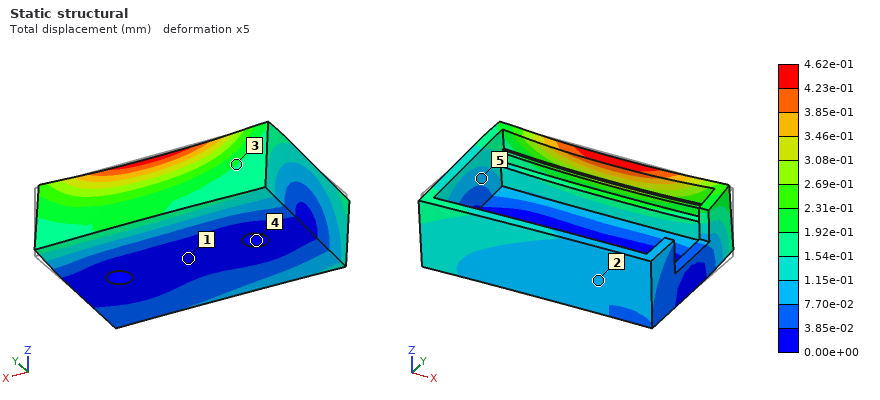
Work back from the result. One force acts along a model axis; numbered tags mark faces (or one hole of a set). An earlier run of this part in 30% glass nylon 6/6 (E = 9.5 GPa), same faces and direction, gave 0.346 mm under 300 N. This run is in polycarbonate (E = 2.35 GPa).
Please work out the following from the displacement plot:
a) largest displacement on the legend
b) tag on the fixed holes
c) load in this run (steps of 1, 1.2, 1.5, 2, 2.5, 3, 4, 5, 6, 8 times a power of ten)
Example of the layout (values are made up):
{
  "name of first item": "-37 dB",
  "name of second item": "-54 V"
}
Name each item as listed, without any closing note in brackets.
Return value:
{
  "largest displacement on the legend": "4.62e-01 mm",
  "tag on the fixed holes": "4",
  "load in this run": "100 N"
}
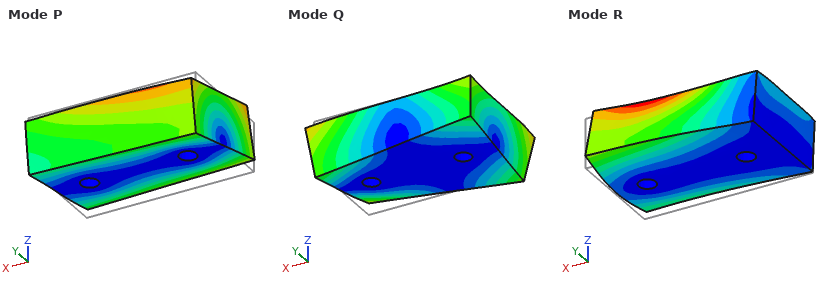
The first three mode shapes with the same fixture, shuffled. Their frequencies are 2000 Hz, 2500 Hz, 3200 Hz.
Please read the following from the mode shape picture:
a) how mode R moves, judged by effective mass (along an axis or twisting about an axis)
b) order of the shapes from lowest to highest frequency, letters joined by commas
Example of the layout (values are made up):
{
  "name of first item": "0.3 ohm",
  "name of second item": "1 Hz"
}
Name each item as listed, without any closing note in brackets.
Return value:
{
  "how mode R moves, judged by effective mass": "along Z",
  "order of the shapes from lowest to highest frequency, letters joined by commas": "P, Q, R"
}
